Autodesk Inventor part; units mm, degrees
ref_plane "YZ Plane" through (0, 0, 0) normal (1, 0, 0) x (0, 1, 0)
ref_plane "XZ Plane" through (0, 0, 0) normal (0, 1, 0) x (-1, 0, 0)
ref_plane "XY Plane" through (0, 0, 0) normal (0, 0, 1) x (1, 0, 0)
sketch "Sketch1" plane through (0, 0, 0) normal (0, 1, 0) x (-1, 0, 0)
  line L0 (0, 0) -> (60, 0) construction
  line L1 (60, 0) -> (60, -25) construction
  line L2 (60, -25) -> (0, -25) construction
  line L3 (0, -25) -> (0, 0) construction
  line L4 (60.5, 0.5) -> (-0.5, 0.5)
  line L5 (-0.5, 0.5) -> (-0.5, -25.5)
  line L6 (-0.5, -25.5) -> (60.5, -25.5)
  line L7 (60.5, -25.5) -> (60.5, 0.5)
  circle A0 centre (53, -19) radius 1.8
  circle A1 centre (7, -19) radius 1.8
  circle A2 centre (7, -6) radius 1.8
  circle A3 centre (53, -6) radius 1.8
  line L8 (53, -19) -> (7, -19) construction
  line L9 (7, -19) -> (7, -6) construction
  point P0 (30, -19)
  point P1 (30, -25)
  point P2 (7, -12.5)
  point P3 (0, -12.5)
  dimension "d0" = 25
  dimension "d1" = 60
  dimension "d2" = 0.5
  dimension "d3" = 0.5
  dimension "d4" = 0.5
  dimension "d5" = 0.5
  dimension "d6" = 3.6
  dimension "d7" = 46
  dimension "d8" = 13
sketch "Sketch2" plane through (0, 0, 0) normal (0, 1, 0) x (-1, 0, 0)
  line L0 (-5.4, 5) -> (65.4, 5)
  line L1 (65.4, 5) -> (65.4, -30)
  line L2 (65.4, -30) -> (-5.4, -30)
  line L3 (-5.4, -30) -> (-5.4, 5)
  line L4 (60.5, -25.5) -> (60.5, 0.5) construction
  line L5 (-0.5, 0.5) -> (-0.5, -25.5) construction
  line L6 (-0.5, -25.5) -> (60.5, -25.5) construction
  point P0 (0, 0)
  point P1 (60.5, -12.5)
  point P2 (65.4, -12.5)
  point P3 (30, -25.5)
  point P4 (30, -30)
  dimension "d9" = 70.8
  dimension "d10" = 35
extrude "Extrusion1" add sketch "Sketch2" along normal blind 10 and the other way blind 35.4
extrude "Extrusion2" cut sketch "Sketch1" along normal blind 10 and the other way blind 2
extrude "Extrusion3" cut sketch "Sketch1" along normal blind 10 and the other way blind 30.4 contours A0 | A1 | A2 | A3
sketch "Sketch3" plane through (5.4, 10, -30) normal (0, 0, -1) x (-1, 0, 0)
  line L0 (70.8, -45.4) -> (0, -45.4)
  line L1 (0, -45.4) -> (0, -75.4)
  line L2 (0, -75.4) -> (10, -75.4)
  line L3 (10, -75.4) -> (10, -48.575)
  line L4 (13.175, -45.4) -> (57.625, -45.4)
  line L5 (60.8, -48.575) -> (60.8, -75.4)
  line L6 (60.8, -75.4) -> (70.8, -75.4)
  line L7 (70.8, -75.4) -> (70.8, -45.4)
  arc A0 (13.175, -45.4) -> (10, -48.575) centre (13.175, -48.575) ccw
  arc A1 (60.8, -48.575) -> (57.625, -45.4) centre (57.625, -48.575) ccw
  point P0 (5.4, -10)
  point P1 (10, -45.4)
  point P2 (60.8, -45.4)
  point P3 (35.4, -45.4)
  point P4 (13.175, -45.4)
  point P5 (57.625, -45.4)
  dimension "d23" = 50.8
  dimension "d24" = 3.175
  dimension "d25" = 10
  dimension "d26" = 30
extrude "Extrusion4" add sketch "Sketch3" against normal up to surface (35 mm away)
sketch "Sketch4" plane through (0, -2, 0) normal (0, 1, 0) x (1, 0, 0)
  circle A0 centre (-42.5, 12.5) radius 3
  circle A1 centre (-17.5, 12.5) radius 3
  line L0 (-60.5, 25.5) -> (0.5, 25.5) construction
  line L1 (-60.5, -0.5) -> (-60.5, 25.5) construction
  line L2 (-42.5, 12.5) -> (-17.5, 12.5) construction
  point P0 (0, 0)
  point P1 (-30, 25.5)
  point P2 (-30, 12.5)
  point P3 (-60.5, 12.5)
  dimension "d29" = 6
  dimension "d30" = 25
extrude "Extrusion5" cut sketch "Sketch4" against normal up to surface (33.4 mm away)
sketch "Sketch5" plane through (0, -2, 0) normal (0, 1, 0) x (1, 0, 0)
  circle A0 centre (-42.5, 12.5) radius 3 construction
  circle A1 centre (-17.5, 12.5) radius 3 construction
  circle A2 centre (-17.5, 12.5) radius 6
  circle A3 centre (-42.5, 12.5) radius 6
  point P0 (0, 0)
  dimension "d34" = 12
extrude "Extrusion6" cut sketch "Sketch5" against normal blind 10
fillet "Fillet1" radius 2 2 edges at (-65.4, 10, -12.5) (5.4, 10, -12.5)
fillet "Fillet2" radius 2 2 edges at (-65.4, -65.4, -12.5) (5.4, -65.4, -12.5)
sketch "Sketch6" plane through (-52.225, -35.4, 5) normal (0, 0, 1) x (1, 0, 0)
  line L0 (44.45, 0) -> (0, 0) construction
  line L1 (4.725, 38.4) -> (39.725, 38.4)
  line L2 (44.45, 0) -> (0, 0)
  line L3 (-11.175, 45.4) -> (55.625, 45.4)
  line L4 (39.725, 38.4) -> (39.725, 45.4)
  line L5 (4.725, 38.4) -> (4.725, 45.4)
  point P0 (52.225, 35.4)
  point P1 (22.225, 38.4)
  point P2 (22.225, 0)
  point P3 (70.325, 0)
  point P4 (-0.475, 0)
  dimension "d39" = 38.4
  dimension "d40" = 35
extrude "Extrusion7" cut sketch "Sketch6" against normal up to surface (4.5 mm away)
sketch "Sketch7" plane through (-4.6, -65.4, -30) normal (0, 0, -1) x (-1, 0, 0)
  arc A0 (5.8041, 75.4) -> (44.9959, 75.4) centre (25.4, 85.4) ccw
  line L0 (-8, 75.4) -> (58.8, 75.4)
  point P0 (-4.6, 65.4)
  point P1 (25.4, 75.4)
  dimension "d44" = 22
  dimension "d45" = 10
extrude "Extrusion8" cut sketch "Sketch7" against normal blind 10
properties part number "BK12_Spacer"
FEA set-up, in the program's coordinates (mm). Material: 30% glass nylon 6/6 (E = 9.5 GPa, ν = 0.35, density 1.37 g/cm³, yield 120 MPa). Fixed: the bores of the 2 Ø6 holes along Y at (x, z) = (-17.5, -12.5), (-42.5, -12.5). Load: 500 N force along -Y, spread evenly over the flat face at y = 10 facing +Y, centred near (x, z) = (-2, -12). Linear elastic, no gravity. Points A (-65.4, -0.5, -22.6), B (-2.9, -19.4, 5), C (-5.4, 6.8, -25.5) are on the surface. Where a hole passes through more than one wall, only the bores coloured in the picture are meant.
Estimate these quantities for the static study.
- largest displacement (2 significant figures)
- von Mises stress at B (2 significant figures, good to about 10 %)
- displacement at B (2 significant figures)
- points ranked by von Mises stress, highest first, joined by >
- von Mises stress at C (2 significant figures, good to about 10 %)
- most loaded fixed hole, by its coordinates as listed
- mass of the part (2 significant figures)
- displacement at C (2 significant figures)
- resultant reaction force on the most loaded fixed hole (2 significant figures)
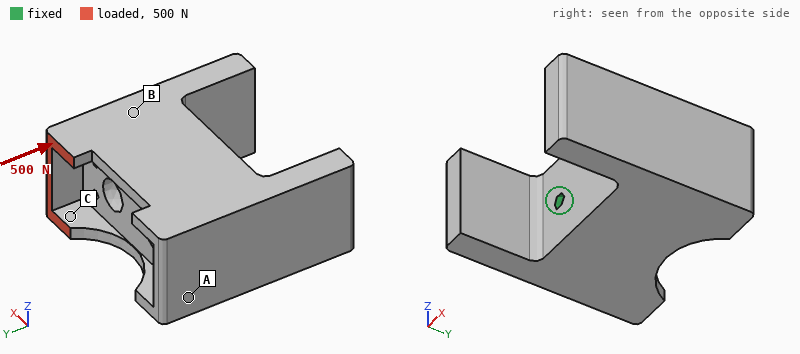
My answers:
13 µm
0.86 MPa
5.2 µm
C > B > A
2.2 MPa
(-17.5, -12.5)
150 g
10 µm
580 N
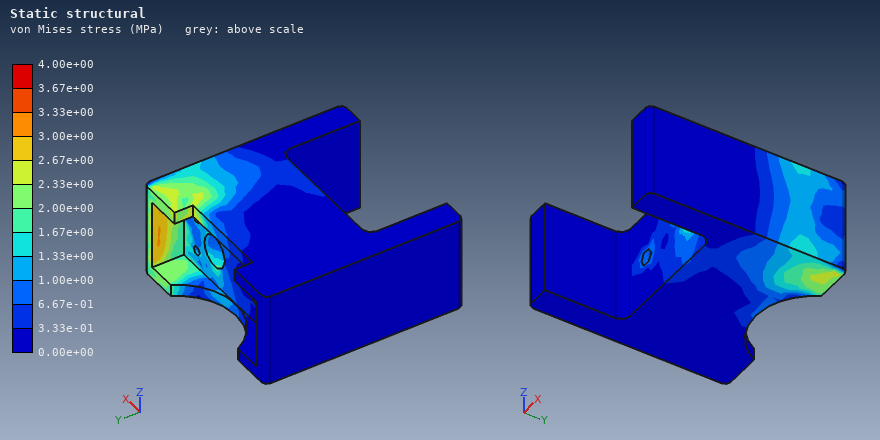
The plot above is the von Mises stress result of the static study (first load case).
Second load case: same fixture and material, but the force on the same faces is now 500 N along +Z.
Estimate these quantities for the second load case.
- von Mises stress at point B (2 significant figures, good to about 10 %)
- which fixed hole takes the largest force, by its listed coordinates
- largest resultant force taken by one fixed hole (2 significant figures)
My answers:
2.7 MPa
(-17.5, -12.5)
720 N
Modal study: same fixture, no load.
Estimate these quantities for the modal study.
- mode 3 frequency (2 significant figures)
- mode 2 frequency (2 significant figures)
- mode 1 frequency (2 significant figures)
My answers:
4100 Hz
3300 Hz
3200 Hz
